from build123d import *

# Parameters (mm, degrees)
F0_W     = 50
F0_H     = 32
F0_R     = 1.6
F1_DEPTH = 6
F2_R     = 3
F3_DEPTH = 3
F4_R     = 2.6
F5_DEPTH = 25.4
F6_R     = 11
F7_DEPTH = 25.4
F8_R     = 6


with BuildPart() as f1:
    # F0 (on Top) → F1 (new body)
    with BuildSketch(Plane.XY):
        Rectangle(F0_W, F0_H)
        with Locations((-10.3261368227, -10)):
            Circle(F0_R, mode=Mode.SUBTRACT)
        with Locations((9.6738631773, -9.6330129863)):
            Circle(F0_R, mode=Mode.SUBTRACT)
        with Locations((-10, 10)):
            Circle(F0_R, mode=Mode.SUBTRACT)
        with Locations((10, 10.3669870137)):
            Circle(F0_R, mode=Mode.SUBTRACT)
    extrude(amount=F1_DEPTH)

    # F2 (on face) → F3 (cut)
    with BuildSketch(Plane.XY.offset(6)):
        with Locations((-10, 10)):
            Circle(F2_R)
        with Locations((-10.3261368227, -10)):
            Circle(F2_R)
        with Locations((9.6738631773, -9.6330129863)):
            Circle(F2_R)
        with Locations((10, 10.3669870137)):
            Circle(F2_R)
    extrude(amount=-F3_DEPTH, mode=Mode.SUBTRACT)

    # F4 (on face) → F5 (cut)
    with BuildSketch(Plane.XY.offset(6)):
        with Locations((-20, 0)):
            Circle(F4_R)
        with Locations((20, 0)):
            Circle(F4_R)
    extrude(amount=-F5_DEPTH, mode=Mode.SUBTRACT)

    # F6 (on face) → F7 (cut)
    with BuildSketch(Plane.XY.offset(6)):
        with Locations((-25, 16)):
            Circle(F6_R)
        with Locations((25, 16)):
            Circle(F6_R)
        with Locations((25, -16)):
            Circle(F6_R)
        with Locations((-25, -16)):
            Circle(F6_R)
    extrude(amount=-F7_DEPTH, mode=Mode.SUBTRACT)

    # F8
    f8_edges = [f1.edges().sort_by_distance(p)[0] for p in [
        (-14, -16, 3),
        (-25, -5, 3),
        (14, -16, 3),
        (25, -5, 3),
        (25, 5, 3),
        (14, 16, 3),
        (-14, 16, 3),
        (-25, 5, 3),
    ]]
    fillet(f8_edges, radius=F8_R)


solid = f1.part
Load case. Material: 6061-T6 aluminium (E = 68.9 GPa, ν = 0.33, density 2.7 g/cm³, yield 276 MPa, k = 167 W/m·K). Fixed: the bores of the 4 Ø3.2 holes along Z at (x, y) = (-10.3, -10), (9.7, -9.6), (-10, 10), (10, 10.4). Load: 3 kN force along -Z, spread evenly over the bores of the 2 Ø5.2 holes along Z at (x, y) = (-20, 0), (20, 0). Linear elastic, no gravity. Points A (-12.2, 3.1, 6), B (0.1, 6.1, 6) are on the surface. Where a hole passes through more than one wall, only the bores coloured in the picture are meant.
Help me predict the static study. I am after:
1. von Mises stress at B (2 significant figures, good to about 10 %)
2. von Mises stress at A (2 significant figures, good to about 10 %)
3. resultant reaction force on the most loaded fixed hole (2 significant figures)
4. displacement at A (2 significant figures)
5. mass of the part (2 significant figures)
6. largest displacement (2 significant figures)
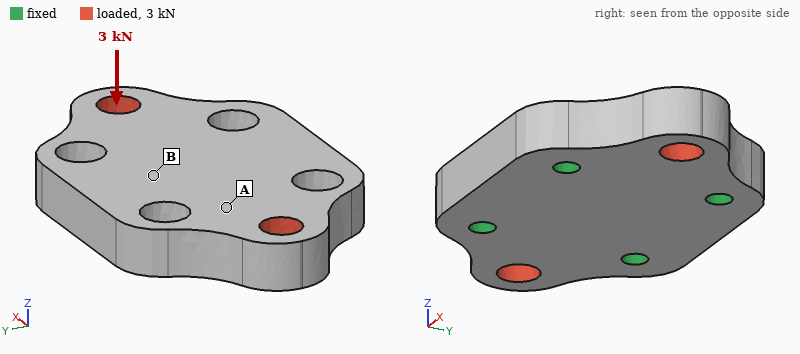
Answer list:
45 MPa
100 MPa
1.3 kN
20 µm
17 g
99 µm
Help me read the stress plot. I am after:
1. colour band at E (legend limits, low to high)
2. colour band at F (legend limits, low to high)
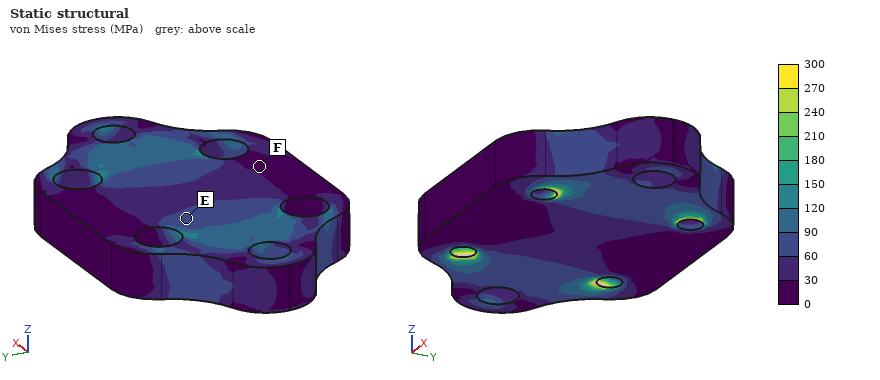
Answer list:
60 to 90 MPa
0 to 30 MPa
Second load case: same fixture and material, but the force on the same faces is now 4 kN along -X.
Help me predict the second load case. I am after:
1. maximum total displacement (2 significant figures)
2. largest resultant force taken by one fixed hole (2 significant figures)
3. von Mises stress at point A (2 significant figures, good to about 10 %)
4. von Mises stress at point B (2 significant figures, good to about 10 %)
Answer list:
13 µm
1.1 kN
24 MPa
11 MPa
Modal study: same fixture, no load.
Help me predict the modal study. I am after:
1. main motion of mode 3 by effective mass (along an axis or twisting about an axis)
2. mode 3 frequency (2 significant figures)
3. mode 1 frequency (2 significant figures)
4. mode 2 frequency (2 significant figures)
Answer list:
along Z
35 kHz
20 kHz
20 kHz
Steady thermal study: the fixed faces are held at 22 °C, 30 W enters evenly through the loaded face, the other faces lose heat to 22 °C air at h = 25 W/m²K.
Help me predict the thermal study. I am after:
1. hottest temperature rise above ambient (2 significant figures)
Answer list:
16 K
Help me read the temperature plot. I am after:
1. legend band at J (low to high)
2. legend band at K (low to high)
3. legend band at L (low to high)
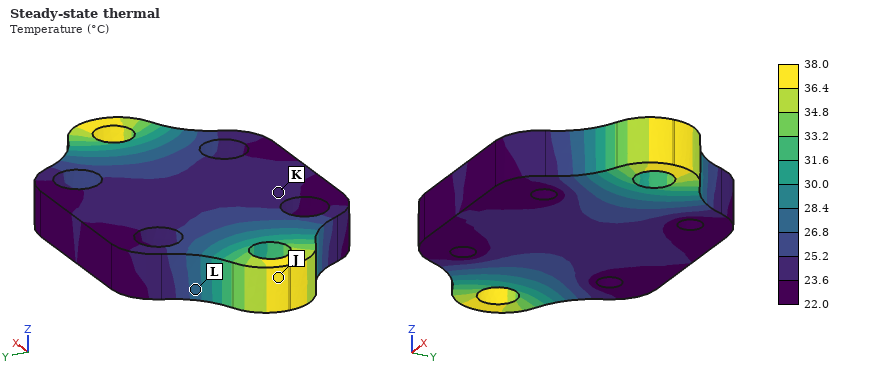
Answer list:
36.4 to 38.0 °C
23.6 to 25.2 °C
26.8 to 28.4 °C
